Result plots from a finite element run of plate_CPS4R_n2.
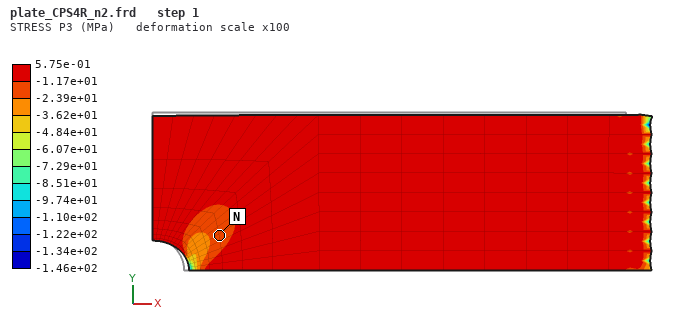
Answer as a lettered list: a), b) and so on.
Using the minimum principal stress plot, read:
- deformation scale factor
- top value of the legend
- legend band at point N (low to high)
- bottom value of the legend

a) 100
b) 5.75e-01 MPa
c) -2.39e+01 to -1.17e+01 MPa
d) -1.46e+02 MPa
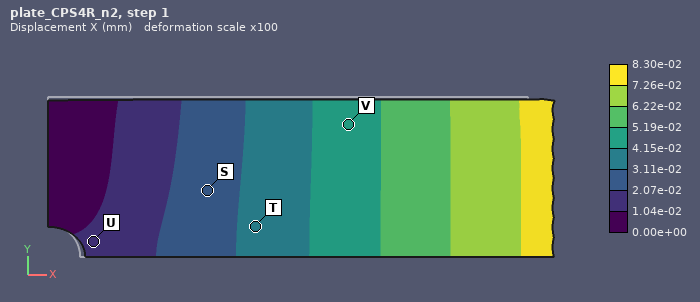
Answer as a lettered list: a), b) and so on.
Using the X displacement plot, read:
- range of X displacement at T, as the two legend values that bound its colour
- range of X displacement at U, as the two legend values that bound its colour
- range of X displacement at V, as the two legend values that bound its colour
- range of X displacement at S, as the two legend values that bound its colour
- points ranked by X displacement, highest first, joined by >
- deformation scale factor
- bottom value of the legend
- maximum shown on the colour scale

a) 3.11e-02 to 4.15e-02 mm
b) 1.04e-02 to 2.07e-02 mm
c) 4.15e-02 to 5.19e-02 mm
d) 2.07e-02 to 3.11e-02 mm
e) V > T > S > U
f) 100
g) 0.00e+00 mm
h) 8.30e-02 mm
